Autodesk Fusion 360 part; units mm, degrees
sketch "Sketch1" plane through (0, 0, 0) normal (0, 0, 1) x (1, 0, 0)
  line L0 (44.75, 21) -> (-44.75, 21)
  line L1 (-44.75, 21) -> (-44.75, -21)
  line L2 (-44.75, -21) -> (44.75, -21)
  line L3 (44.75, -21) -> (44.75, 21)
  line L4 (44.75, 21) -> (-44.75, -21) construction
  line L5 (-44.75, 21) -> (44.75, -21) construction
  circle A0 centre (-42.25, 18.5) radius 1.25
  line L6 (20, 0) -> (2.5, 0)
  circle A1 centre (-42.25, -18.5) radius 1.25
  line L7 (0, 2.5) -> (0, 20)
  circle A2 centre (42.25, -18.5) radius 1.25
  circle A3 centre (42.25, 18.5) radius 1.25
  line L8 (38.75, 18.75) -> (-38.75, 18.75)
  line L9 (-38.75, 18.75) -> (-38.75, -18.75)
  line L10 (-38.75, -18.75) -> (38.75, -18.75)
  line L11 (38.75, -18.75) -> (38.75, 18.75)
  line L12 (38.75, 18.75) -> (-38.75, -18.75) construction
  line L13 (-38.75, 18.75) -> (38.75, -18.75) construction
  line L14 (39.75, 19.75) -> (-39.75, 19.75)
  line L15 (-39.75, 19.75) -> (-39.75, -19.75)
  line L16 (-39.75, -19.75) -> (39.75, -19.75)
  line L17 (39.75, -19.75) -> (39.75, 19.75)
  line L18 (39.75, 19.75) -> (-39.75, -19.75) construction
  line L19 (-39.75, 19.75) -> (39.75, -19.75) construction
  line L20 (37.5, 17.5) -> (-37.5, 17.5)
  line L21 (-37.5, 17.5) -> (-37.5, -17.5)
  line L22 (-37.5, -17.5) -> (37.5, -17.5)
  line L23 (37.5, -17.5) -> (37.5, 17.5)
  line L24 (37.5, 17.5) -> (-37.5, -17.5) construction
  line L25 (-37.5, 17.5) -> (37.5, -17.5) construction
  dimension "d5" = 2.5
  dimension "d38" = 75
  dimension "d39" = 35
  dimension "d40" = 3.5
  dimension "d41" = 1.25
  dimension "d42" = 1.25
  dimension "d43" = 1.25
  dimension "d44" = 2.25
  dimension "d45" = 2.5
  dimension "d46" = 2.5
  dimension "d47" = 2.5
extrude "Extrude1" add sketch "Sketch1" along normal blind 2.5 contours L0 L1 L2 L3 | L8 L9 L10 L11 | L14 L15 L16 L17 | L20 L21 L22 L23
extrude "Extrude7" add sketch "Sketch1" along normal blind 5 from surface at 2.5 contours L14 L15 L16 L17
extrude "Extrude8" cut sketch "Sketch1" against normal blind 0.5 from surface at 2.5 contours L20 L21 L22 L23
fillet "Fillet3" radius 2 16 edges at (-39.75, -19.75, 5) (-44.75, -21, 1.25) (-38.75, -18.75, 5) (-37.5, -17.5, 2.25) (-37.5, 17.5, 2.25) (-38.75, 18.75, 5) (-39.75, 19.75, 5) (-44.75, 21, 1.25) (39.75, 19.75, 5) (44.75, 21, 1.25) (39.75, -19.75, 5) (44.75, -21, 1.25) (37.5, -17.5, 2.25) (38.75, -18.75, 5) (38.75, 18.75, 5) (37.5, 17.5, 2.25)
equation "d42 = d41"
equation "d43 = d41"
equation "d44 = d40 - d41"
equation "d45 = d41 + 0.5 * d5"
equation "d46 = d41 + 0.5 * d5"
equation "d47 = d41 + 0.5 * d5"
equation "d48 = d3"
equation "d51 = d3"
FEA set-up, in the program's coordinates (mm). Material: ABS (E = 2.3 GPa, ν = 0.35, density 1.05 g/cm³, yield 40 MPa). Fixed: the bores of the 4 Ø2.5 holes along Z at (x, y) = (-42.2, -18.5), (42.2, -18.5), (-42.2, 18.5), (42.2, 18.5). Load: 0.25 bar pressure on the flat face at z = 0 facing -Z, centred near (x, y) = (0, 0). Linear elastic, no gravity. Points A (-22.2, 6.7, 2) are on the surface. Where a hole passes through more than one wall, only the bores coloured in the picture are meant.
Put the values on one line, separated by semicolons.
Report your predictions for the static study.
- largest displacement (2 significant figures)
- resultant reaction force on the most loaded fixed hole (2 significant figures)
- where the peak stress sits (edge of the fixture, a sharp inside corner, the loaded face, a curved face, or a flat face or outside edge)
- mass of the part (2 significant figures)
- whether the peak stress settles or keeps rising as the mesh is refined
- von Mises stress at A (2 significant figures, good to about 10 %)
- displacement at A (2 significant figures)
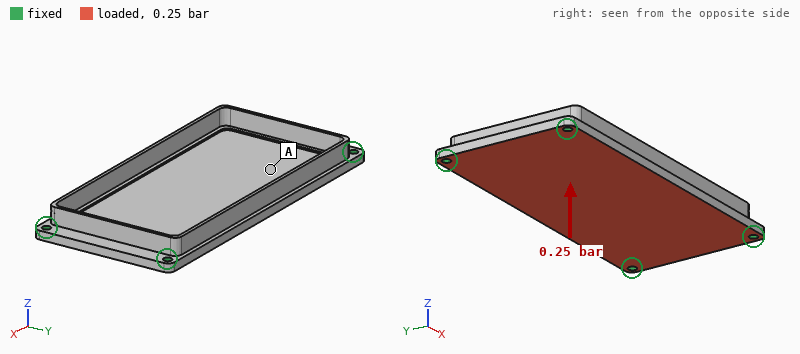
0.90 mm; 25 N; edge of the fixture; 9.7 g; keeps rising; 2.6 MPa; 0.55 mm
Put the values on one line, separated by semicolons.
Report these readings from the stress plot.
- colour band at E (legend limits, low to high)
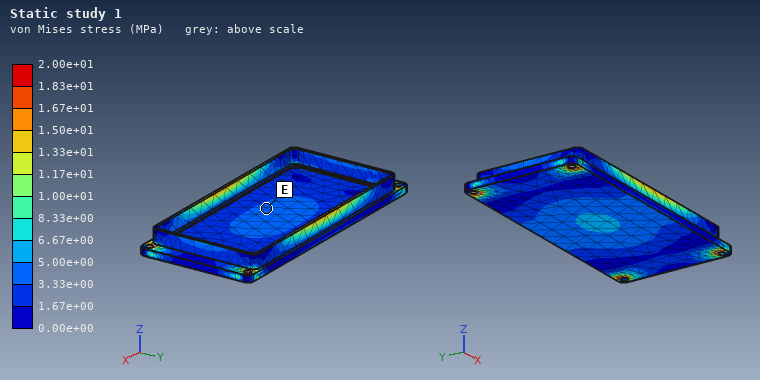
3.33e+00 to 5.00e+00 MPa
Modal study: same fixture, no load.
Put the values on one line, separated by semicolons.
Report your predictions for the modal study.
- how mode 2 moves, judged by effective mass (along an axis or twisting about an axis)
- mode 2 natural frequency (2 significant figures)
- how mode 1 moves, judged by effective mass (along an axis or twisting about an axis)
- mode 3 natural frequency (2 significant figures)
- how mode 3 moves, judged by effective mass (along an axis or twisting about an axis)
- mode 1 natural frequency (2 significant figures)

twisting about X; 990 Hz; along Z; 1700 Hz; twisting about Y; 640 Hz
